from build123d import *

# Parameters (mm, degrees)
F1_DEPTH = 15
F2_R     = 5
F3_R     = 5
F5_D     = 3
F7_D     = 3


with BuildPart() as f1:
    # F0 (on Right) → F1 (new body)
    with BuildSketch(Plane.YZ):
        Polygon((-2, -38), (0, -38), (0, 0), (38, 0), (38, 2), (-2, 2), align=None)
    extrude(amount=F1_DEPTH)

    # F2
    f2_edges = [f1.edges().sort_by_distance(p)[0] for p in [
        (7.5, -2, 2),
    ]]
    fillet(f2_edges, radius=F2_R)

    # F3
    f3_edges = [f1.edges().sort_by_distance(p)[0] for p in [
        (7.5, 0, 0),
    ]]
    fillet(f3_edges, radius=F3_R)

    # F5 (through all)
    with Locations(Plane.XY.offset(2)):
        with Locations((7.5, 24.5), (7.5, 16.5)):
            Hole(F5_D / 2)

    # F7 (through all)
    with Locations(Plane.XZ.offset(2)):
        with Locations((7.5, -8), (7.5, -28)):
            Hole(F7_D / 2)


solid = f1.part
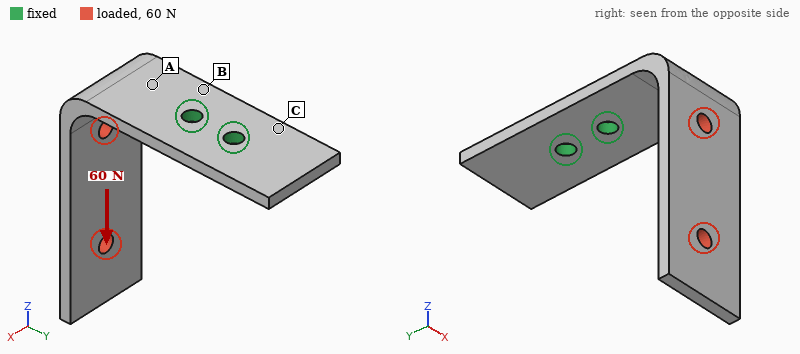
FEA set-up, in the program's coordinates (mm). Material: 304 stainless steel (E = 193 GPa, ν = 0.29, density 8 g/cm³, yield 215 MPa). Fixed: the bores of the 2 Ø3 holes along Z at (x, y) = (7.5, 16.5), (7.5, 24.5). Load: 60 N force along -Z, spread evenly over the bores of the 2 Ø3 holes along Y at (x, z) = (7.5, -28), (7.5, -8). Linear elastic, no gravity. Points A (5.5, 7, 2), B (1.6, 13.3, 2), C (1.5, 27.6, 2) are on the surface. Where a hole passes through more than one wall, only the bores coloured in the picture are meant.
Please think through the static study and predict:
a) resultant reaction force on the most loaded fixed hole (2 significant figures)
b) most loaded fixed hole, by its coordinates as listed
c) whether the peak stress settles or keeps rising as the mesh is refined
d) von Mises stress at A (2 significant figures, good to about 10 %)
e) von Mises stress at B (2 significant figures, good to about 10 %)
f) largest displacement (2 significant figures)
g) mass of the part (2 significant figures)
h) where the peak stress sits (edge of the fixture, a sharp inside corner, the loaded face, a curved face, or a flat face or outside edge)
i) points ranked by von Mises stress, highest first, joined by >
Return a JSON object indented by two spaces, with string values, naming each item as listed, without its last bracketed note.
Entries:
{
  "resultant reaction force on the most loaded fixed hole": "95 N",
  "most loaded fixed hole, by its coordinates as listed": "(7.5, 16.5)",
  "whether the peak stress settles or keeps rising as the mesh is refined": "keeps rising",
  "von Mises stress at A": "43 MPa",
  "von Mises stress at B": "69 MPa",
  "largest displacement": "0.18 mm",
  "mass of the part": "18 g",
  "where the peak stress sits": "edge of the fixture",
  "points ranked by von Mises stress, highest first, joined by >": "B > A > C"
}
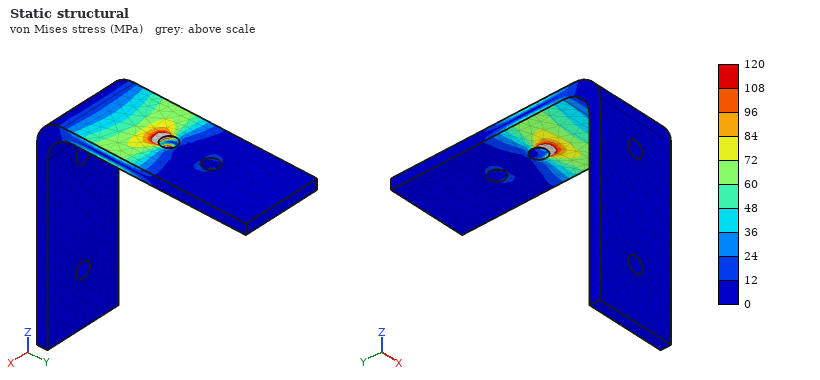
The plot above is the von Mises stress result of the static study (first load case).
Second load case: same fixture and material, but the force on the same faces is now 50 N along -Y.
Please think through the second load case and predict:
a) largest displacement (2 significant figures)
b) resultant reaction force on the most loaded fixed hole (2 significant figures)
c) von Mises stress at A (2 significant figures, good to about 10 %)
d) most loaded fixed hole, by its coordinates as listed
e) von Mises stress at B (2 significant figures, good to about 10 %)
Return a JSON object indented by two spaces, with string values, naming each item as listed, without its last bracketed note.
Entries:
{
  "largest displacement": "0.41 mm",
  "resultant reaction force on the most loaded fixed hole": "51 N",
  "von Mises stress at A": "83 MPa",
  "most loaded fixed hole, by its coordinates as listed": "(7.5, 16.5)",
  "von Mises stress at B": "79 MPa"
}
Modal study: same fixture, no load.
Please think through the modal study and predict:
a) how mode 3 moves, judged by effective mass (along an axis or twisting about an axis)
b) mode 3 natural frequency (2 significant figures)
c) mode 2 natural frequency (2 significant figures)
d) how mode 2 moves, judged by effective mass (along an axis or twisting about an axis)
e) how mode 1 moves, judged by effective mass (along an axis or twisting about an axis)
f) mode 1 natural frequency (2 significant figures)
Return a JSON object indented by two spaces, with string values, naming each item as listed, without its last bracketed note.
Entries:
{
  "how mode 3 moves, judged by effective mass": "along Z",
  "mode 3 natural frequency": "2500 Hz",
  "mode 2 natural frequency": "1100 Hz",
  "how mode 2 moves, judged by effective mass": "along X",
  "how mode 1 moves, judged by effective mass": "along Y",
  "mode 1 natural frequency": "680 Hz"
}
